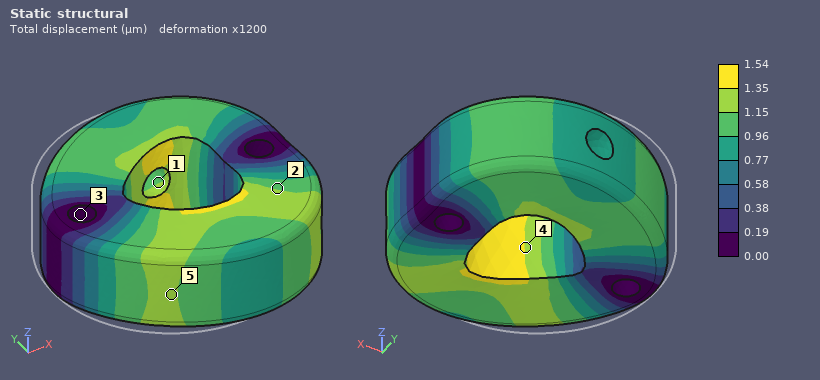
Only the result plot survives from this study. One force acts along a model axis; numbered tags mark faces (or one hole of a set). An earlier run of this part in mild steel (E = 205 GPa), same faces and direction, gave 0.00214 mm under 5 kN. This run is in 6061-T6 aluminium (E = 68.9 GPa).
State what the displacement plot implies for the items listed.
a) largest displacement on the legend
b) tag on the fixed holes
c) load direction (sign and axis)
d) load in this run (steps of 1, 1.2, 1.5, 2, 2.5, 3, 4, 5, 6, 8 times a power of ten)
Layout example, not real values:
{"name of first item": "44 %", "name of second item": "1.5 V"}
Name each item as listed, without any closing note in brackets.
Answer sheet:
{"largest displacement on the legend": "1.54 µm", "tag on the fixed holes": "3", "load direction": "+X", "load in this run": "1.2 kN"}
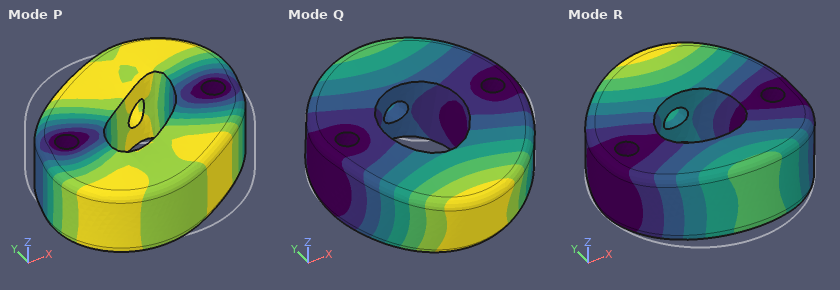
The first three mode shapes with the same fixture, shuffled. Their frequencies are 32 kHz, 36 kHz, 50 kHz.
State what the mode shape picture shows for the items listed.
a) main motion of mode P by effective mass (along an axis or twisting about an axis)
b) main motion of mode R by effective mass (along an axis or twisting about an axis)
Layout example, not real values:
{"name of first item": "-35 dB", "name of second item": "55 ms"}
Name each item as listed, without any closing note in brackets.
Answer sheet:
{"main motion of mode P by effective mass": "twisting about Z", "main motion of mode R by effective mass": "along Z"}
